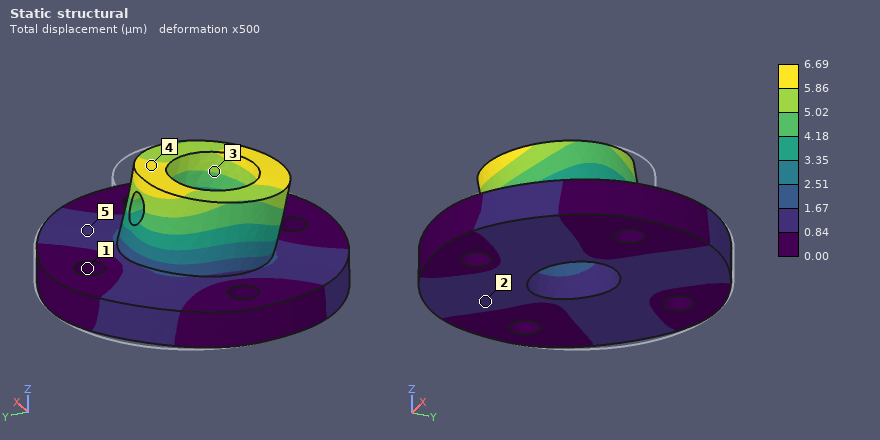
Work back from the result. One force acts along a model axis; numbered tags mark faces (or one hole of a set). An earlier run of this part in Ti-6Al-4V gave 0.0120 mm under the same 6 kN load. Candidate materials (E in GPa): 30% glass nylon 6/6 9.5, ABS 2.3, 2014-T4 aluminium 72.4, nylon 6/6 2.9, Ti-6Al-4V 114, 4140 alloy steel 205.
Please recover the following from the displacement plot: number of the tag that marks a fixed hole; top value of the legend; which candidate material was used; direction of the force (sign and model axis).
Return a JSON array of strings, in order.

["1", "6.69 µm", "4140 alloy steel", "-Y"]
